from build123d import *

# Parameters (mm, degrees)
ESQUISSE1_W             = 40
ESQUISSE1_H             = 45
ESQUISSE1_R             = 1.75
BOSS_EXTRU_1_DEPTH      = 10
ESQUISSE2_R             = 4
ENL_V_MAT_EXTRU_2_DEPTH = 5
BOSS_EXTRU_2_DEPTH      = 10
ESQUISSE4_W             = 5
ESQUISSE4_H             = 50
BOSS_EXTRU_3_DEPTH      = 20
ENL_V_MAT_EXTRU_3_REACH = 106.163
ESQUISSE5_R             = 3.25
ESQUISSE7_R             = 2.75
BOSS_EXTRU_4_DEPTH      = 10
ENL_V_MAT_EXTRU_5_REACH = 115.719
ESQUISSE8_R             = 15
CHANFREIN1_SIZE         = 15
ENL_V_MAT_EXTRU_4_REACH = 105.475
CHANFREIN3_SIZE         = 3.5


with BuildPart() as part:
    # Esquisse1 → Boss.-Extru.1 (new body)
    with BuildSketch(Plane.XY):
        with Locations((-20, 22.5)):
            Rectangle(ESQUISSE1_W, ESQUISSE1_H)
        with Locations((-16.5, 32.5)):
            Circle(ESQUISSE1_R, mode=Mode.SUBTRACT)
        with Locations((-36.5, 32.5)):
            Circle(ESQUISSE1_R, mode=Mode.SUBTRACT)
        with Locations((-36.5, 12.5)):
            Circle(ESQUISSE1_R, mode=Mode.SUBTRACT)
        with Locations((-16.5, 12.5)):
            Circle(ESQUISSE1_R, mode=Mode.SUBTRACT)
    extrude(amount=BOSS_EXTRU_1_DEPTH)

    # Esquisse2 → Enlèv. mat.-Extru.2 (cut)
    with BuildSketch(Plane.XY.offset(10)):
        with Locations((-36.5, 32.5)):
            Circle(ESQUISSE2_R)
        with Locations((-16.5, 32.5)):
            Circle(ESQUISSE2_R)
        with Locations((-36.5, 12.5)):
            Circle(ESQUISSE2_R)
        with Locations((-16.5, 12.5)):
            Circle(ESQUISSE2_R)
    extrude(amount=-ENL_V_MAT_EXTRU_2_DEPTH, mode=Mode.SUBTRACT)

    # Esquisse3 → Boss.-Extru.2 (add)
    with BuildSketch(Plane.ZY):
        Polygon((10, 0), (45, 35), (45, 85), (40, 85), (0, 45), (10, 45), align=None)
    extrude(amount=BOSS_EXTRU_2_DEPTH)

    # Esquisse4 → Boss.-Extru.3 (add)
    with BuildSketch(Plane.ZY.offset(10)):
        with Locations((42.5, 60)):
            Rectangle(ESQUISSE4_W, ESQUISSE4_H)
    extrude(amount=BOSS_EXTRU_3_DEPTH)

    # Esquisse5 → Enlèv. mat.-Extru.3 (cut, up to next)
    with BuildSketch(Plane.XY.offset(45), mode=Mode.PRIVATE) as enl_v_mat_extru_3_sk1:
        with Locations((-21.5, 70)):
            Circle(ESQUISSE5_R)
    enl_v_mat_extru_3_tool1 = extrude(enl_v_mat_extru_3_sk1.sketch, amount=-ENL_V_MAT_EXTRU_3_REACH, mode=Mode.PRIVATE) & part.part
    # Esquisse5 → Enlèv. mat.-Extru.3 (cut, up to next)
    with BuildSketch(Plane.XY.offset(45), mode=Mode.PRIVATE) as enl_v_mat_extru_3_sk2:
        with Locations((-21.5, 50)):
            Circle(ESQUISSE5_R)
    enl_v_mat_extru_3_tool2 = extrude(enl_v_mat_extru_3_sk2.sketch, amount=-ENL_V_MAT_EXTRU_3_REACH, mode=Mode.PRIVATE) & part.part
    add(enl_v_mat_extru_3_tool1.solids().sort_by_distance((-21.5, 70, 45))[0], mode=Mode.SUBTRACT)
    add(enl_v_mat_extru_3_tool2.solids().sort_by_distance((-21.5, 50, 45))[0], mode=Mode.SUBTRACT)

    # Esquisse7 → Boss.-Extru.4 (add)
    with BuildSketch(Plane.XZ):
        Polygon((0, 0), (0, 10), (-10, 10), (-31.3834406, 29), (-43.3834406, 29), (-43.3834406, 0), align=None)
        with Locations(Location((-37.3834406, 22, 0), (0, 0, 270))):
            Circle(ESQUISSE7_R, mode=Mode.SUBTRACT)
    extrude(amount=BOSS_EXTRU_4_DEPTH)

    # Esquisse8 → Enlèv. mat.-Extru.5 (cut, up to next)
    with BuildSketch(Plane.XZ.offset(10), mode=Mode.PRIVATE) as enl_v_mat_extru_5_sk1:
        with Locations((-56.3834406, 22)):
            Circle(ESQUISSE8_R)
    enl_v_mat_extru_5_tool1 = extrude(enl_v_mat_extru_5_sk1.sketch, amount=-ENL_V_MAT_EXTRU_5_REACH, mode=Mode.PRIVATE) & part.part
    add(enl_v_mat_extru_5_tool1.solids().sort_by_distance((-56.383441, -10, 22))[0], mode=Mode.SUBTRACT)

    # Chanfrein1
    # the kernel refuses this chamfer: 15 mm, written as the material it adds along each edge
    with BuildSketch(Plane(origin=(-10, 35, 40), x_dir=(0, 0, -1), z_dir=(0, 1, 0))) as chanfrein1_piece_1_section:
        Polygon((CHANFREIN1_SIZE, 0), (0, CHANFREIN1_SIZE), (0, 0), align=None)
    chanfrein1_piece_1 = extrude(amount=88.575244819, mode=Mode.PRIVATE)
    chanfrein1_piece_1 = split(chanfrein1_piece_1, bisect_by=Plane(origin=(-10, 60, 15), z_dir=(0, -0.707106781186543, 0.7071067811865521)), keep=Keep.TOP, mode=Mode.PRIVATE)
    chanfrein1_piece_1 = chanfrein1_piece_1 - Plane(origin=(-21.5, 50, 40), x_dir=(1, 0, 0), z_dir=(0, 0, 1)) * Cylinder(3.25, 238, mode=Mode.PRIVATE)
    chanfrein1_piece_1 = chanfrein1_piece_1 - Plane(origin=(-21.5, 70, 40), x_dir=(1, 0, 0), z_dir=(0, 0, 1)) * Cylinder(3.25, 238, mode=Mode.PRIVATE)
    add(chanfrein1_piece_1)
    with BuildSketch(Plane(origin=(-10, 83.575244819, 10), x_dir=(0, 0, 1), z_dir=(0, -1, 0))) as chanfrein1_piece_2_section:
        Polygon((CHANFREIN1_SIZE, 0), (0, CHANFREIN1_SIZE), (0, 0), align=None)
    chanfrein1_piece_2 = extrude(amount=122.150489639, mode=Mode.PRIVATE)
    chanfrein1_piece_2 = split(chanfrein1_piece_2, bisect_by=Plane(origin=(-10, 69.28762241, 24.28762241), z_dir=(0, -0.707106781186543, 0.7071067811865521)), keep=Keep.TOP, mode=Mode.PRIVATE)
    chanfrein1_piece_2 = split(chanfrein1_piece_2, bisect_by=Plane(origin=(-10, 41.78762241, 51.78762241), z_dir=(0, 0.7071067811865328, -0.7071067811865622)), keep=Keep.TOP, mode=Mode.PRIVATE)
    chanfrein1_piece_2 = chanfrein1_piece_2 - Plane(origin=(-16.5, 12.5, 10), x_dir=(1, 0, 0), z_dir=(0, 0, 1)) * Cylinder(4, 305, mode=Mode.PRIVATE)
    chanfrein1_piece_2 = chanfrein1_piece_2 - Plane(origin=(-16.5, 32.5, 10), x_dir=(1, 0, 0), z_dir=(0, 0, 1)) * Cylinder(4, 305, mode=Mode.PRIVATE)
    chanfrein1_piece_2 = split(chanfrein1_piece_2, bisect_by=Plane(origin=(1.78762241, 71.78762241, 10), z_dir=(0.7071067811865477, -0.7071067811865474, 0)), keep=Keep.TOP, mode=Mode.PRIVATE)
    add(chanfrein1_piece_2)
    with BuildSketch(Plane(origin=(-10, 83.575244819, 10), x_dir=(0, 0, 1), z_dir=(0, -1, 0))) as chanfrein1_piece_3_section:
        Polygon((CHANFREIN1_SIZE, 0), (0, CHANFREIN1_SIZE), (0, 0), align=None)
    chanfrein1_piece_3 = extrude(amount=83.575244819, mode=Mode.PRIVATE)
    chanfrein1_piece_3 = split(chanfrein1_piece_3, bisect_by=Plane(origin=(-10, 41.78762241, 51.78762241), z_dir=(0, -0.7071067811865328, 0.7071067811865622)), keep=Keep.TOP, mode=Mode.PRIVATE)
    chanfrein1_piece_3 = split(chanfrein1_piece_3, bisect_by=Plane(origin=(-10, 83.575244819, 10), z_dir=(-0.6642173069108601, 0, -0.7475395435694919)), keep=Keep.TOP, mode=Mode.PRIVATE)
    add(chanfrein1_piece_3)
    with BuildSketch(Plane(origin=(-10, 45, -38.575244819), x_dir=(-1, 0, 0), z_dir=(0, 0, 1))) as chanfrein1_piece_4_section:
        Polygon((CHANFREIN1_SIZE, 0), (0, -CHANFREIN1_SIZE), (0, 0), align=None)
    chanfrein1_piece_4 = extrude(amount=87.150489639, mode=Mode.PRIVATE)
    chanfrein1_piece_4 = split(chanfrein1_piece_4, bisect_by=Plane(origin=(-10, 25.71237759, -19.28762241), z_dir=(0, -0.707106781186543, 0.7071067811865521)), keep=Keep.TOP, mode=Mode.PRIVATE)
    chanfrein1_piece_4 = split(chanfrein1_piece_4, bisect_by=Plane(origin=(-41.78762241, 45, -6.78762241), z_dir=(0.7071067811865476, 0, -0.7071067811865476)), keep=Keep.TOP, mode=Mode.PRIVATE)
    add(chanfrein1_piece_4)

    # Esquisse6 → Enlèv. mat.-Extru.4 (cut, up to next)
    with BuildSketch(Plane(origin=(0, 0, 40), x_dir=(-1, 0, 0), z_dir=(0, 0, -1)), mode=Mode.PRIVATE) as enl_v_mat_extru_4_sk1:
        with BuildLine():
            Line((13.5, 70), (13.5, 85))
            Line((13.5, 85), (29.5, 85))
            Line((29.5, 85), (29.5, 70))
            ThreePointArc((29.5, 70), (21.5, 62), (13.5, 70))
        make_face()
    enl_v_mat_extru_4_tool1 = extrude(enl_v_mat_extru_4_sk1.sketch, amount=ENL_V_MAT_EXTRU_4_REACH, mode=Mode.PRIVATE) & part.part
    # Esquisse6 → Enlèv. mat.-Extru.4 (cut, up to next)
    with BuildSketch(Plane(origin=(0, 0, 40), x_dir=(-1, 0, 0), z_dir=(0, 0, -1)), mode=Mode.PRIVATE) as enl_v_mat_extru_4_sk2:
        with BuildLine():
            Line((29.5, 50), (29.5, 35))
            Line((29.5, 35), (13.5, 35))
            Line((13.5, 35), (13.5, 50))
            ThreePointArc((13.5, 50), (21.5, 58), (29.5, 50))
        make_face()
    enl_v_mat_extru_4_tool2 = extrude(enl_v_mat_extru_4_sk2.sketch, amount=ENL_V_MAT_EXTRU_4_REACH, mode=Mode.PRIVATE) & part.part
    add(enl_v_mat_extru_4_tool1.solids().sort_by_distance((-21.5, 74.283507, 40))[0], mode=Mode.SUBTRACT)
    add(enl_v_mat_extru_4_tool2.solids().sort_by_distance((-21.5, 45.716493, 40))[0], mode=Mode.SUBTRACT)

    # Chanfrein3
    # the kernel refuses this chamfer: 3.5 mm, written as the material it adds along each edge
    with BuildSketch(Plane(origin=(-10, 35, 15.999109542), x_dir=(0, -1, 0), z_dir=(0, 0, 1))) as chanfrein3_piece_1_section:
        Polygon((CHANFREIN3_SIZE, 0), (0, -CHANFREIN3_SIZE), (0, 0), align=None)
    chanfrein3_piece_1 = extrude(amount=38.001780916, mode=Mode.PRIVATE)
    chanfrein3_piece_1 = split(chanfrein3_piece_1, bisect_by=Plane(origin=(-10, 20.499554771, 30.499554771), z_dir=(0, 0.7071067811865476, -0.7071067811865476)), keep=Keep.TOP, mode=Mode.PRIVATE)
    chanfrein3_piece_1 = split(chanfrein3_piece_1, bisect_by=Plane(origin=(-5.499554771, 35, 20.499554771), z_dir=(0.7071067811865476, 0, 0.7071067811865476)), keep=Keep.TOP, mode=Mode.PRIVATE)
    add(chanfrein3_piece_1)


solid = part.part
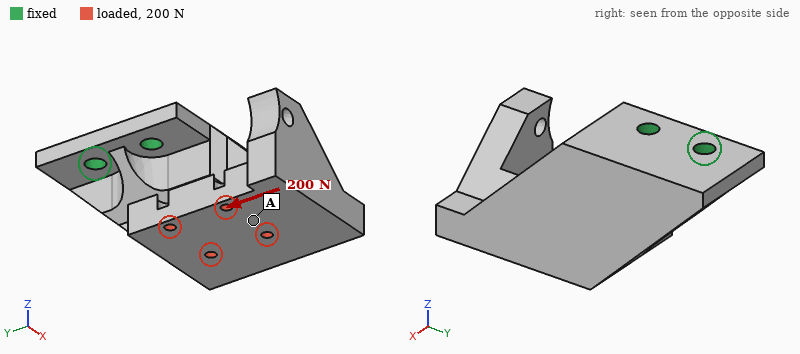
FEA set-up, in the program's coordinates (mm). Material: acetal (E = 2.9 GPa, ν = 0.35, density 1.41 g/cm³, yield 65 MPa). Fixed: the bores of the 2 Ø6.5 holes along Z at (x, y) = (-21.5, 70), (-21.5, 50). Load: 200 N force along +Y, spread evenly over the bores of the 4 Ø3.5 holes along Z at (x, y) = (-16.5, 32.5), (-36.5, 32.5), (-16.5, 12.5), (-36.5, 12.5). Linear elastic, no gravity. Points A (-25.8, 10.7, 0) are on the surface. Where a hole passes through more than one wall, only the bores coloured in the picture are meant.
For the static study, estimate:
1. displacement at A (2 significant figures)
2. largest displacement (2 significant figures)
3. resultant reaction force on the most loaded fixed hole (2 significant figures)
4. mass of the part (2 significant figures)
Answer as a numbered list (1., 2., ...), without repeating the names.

1. 0.68 mm
2. 0.91 mm
3. 350 N
4. 81 g
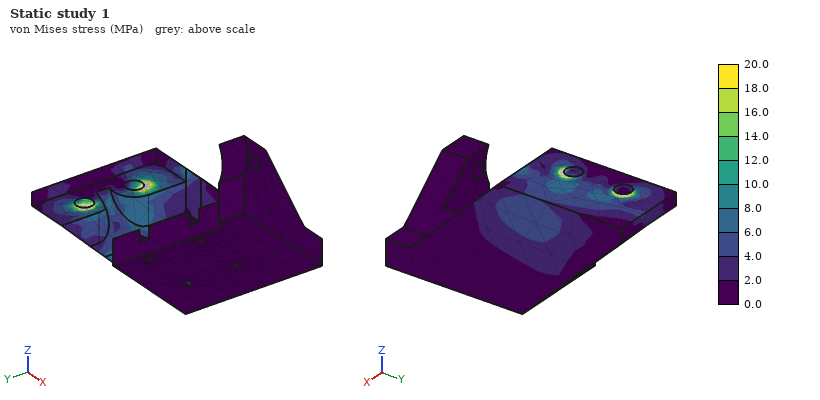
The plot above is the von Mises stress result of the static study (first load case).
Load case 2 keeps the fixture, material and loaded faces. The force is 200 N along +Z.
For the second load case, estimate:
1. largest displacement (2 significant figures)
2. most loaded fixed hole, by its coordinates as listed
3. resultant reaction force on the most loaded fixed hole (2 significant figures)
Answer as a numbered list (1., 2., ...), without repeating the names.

1. 1.1 mm
2. (-21.5, 50)
3. 400 N
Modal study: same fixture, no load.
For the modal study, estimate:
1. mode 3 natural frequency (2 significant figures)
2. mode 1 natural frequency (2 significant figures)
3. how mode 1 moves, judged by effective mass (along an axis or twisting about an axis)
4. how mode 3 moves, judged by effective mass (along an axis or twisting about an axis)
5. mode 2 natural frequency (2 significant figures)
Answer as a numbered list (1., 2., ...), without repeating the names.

1. 800 Hz
2. 250 Hz
3. along X
4. along Z
5. 380 Hz
